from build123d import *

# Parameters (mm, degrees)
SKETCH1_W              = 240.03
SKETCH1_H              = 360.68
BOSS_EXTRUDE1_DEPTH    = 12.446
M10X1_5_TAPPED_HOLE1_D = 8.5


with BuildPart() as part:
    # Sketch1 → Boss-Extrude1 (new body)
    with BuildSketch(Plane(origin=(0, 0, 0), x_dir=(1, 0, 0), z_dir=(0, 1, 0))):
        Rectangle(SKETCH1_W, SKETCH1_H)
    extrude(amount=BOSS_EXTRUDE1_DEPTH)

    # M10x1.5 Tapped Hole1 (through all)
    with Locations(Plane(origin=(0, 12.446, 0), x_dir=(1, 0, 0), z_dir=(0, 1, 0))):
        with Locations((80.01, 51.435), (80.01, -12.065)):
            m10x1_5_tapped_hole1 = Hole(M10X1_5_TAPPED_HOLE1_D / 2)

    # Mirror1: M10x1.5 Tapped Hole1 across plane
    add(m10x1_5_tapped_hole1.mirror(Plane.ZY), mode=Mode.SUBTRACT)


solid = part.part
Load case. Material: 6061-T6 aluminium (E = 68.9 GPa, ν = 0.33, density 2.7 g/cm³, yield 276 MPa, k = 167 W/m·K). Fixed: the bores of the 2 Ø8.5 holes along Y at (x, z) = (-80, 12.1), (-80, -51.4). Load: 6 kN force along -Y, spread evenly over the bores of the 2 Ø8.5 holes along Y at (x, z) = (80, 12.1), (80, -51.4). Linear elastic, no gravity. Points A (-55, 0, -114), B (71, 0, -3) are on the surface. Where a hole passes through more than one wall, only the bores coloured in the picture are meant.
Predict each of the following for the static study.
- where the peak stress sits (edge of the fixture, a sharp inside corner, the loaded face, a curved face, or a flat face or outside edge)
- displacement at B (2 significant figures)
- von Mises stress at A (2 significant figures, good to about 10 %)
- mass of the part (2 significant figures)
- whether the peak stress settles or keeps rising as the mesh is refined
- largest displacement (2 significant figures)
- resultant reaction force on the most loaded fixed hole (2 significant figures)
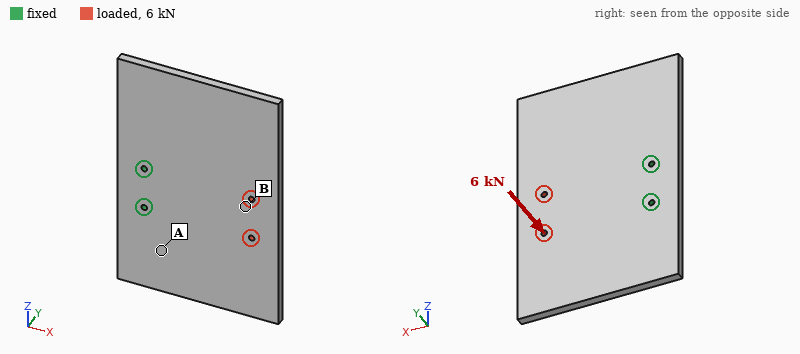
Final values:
edge of the fixture
3.5 mm
69 MPa
2.9 kg
keeps rising
5.0 mm
3.0 kN
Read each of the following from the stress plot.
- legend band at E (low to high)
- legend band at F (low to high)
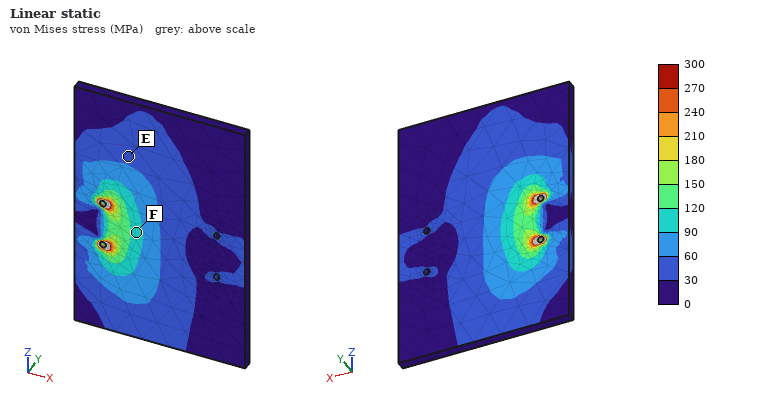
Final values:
30 to 60 MPa
90 to 120 MPa
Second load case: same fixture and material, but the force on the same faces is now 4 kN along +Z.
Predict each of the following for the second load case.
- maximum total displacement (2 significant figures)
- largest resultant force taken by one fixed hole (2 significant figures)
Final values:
0.11 mm
9.6 kN
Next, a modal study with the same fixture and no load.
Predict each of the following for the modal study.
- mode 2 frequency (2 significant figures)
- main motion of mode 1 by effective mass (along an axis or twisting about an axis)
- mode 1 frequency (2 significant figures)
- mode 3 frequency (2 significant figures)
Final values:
230 Hz
along Y
180 Hz
430 Hz
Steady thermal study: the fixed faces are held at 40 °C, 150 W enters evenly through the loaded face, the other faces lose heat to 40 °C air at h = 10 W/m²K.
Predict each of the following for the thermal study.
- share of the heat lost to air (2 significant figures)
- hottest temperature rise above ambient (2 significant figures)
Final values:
29 %
55 K
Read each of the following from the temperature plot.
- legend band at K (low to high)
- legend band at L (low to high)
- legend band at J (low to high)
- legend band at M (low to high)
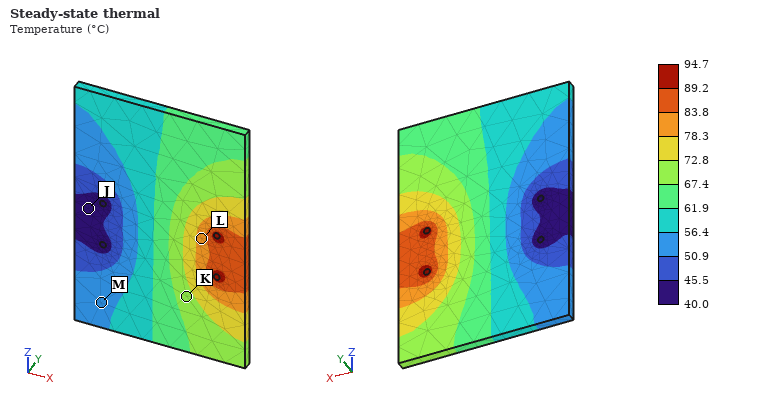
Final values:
67.4 to 72.8 °C
78.3 to 83.8 °C
40.0 to 45.5 °C
50.9 to 56.4 °C
